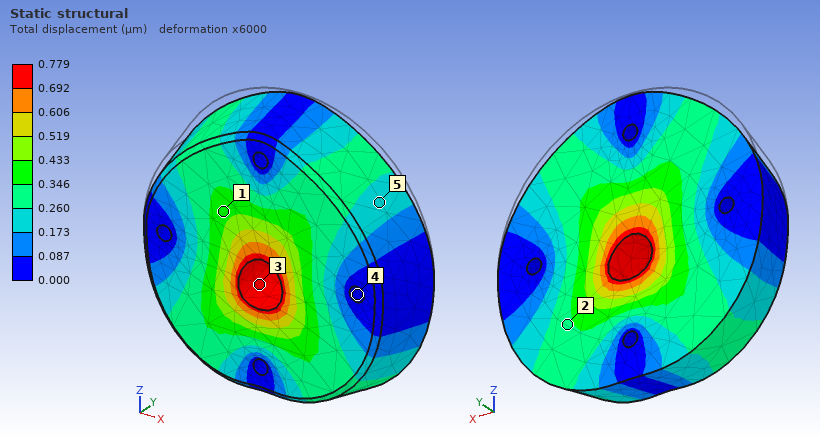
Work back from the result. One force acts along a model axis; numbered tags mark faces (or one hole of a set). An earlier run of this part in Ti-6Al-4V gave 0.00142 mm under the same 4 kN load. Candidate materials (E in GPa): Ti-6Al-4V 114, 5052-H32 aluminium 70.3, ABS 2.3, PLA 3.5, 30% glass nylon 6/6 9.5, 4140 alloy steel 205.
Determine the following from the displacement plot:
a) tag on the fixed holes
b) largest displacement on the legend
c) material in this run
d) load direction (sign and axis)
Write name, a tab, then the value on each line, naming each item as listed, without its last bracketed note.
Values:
tag on the fixed holes	4
largest displacement on the legend	0.779 µm
material in this run	4140 alloy steel
load direction	-Z
